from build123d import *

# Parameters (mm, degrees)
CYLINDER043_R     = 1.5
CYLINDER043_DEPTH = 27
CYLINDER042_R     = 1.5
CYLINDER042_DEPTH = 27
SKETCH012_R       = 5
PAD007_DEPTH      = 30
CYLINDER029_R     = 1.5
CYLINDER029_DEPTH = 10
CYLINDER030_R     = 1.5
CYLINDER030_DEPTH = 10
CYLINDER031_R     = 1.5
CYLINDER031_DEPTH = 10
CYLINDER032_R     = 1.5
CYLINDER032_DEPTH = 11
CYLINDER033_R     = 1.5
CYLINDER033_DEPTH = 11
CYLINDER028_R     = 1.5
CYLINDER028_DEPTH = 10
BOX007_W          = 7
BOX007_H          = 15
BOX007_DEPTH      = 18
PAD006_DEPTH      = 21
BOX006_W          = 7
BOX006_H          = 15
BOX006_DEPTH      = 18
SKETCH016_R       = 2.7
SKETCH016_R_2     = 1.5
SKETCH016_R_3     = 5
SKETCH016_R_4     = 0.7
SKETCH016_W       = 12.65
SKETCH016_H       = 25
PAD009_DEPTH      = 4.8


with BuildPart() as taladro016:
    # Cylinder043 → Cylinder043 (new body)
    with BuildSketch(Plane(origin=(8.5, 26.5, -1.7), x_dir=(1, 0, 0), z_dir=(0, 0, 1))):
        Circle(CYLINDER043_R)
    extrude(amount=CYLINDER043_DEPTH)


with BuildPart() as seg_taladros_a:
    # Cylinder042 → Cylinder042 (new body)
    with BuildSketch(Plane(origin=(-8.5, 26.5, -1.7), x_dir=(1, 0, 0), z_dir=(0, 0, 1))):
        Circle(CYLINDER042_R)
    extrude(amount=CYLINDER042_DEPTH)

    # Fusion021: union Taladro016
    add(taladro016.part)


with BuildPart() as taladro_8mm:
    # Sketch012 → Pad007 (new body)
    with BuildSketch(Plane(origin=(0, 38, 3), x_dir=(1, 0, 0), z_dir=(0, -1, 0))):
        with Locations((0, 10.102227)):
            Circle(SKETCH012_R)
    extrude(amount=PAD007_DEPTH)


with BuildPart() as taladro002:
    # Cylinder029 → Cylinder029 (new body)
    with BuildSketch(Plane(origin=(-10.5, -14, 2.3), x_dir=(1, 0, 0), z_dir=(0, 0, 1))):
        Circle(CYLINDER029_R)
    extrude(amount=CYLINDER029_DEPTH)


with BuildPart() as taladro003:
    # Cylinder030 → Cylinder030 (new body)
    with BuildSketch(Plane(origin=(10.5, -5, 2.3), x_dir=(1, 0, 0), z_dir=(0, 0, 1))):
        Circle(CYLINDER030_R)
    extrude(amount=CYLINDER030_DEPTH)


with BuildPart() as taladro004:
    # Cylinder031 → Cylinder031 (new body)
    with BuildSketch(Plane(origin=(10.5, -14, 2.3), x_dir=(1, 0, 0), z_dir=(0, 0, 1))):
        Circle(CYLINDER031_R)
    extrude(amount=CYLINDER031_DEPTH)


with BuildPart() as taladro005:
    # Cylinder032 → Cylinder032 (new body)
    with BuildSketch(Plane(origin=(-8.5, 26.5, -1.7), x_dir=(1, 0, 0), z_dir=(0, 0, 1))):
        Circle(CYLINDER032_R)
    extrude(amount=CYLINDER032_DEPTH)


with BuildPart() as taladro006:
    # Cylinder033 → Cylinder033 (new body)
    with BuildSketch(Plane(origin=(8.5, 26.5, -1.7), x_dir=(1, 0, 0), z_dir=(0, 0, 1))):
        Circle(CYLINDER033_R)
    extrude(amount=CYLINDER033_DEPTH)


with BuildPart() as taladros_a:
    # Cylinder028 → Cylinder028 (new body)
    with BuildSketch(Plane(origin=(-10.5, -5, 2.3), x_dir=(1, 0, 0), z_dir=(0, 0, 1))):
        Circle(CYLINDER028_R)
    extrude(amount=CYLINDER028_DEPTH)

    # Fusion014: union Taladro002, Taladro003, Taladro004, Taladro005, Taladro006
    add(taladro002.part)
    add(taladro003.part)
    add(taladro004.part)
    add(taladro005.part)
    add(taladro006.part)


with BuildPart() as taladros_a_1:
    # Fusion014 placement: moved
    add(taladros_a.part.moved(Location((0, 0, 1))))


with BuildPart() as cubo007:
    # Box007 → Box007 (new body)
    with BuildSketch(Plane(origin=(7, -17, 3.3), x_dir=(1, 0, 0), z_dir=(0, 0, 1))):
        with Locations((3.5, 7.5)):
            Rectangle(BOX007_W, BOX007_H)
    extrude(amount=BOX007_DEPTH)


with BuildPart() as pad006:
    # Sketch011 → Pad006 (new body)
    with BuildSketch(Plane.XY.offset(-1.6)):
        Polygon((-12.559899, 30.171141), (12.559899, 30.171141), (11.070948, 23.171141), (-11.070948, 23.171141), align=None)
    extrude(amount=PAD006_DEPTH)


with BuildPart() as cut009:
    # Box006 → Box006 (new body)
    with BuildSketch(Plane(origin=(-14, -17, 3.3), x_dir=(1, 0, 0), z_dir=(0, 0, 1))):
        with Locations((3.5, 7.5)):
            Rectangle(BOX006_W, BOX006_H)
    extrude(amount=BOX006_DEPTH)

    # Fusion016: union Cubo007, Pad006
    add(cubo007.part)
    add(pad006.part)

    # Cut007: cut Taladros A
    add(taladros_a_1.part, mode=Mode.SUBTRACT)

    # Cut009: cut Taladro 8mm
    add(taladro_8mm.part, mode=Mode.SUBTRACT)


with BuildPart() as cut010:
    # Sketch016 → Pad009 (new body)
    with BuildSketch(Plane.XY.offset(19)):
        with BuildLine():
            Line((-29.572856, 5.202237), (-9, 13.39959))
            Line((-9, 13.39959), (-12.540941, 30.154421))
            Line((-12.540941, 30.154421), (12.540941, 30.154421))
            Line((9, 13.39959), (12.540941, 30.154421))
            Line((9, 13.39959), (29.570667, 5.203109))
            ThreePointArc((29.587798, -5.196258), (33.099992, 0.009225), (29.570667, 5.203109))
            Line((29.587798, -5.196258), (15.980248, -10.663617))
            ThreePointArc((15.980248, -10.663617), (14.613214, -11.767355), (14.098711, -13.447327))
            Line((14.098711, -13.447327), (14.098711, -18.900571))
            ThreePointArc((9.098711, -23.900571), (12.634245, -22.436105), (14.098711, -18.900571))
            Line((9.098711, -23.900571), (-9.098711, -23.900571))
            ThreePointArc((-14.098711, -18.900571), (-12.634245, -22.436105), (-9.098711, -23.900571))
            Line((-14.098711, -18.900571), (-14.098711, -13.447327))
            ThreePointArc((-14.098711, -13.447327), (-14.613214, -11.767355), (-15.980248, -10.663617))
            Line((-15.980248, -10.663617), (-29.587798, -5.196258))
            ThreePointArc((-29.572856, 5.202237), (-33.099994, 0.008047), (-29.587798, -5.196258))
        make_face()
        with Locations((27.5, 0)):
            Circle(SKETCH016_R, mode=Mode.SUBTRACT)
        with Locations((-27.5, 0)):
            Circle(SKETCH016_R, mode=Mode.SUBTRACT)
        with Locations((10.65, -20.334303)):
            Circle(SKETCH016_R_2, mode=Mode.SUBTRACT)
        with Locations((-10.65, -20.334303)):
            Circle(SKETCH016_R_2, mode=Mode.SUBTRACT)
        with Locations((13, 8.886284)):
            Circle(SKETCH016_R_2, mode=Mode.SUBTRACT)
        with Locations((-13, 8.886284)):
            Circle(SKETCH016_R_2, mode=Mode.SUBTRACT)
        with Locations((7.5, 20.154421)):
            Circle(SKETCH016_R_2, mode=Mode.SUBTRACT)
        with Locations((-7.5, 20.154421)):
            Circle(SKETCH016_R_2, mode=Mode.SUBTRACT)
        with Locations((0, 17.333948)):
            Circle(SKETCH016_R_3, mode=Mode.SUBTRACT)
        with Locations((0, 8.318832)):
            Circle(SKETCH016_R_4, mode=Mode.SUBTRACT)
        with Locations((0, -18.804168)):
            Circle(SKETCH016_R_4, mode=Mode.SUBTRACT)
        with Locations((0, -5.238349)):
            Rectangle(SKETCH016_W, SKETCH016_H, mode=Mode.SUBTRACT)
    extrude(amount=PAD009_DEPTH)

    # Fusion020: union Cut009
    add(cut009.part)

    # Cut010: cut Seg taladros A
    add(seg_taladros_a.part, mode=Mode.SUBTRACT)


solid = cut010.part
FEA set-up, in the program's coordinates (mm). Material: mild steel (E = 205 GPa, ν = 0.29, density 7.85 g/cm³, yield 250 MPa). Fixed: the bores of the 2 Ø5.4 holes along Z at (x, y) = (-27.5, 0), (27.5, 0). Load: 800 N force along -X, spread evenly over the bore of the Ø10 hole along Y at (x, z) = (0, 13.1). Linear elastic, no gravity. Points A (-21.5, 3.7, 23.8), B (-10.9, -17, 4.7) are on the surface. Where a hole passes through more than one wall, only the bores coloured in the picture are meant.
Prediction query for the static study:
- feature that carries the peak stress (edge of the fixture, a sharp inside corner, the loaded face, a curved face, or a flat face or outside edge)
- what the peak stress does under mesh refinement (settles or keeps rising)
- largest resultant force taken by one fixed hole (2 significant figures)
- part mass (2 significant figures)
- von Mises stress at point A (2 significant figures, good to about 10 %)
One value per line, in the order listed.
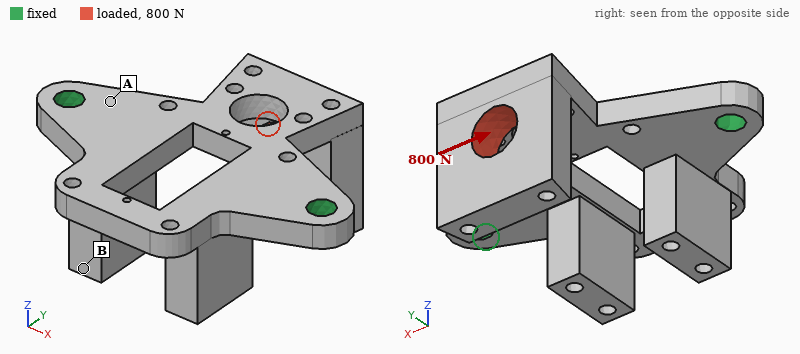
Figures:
a sharp inside corner
keeps rising
660 N
99 g
46 MPa
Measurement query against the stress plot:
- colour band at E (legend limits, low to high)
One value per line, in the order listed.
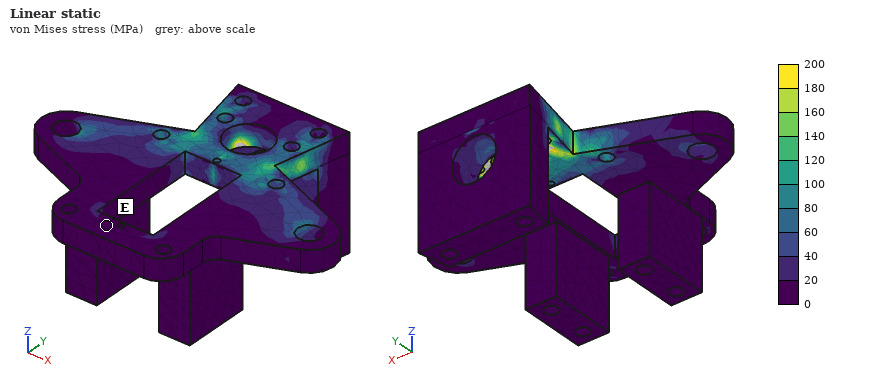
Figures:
0 to 20 MPa
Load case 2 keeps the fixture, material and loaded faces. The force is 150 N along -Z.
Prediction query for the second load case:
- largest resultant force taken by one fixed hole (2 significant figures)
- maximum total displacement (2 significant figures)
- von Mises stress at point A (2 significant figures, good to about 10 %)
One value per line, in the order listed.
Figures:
75 N
81 µm
33 MPa
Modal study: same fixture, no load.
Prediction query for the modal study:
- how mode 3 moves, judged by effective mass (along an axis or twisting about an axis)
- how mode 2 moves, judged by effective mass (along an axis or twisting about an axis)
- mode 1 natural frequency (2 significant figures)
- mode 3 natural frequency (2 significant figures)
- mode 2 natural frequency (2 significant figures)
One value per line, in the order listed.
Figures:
along Z
along X
1400 Hz
3500 Hz
2700 Hz
